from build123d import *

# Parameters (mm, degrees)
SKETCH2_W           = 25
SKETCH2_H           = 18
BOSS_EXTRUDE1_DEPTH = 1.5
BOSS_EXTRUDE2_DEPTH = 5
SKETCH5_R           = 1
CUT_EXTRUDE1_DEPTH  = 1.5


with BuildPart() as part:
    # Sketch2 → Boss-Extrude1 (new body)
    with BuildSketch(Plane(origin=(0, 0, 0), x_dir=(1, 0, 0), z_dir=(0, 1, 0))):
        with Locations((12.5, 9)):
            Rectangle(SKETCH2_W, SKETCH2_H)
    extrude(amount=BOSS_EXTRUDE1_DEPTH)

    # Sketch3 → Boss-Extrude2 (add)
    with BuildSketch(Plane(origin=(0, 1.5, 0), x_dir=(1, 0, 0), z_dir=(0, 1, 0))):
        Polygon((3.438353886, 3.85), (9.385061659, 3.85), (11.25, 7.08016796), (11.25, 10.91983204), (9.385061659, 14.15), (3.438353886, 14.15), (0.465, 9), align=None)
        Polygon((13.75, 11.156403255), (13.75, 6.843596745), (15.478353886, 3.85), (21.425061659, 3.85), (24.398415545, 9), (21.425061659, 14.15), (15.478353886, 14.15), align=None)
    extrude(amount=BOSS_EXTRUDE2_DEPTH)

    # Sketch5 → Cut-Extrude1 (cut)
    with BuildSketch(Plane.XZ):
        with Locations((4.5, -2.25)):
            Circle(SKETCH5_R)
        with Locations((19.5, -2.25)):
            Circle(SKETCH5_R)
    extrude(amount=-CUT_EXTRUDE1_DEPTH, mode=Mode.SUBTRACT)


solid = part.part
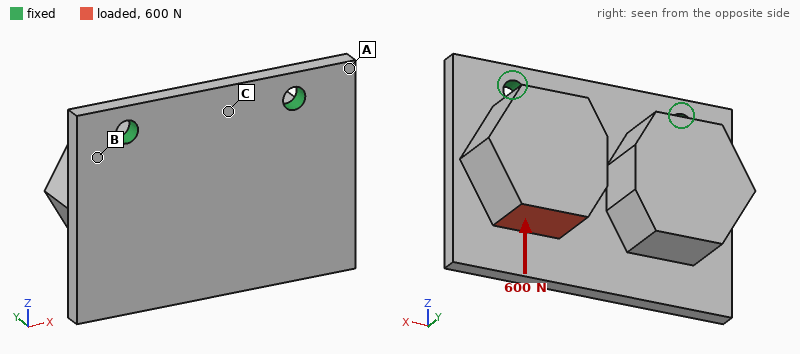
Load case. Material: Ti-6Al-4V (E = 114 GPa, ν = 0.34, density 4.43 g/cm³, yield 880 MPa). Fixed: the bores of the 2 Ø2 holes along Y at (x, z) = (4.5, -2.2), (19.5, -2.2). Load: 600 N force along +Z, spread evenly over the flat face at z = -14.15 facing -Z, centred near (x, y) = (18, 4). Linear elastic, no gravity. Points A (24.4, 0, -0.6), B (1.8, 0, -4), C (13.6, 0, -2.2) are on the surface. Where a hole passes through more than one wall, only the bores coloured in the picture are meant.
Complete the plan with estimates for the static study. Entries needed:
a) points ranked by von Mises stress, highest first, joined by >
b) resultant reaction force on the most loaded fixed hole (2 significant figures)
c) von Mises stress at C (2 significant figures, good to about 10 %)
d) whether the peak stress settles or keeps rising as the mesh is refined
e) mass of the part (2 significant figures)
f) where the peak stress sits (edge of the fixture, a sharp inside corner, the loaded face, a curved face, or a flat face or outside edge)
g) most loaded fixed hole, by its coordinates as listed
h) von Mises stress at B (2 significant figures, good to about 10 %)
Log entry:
B > C > A
550 N
69 MPa
keeps rising
6.9 g
edge of the fixture
(19.5, -2.2)
130 MPa
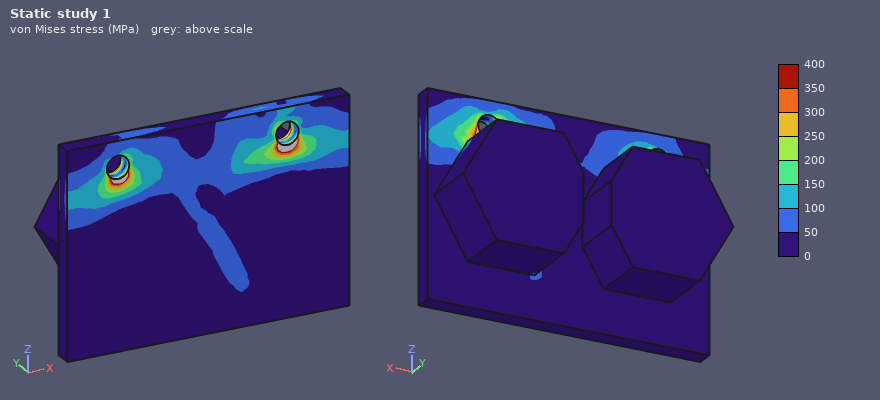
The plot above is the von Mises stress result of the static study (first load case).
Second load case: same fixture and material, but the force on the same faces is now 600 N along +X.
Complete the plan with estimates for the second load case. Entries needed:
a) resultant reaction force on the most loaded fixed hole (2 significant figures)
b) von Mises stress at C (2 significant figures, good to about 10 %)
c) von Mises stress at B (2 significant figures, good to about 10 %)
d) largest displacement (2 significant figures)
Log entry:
560 N
70 MPa
39 MPa
28 µm
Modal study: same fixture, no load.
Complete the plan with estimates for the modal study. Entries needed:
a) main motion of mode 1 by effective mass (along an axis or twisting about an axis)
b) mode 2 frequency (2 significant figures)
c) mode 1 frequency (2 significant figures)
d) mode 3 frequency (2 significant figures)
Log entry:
along Y
11 kHz
4200 Hz
15 kHz
